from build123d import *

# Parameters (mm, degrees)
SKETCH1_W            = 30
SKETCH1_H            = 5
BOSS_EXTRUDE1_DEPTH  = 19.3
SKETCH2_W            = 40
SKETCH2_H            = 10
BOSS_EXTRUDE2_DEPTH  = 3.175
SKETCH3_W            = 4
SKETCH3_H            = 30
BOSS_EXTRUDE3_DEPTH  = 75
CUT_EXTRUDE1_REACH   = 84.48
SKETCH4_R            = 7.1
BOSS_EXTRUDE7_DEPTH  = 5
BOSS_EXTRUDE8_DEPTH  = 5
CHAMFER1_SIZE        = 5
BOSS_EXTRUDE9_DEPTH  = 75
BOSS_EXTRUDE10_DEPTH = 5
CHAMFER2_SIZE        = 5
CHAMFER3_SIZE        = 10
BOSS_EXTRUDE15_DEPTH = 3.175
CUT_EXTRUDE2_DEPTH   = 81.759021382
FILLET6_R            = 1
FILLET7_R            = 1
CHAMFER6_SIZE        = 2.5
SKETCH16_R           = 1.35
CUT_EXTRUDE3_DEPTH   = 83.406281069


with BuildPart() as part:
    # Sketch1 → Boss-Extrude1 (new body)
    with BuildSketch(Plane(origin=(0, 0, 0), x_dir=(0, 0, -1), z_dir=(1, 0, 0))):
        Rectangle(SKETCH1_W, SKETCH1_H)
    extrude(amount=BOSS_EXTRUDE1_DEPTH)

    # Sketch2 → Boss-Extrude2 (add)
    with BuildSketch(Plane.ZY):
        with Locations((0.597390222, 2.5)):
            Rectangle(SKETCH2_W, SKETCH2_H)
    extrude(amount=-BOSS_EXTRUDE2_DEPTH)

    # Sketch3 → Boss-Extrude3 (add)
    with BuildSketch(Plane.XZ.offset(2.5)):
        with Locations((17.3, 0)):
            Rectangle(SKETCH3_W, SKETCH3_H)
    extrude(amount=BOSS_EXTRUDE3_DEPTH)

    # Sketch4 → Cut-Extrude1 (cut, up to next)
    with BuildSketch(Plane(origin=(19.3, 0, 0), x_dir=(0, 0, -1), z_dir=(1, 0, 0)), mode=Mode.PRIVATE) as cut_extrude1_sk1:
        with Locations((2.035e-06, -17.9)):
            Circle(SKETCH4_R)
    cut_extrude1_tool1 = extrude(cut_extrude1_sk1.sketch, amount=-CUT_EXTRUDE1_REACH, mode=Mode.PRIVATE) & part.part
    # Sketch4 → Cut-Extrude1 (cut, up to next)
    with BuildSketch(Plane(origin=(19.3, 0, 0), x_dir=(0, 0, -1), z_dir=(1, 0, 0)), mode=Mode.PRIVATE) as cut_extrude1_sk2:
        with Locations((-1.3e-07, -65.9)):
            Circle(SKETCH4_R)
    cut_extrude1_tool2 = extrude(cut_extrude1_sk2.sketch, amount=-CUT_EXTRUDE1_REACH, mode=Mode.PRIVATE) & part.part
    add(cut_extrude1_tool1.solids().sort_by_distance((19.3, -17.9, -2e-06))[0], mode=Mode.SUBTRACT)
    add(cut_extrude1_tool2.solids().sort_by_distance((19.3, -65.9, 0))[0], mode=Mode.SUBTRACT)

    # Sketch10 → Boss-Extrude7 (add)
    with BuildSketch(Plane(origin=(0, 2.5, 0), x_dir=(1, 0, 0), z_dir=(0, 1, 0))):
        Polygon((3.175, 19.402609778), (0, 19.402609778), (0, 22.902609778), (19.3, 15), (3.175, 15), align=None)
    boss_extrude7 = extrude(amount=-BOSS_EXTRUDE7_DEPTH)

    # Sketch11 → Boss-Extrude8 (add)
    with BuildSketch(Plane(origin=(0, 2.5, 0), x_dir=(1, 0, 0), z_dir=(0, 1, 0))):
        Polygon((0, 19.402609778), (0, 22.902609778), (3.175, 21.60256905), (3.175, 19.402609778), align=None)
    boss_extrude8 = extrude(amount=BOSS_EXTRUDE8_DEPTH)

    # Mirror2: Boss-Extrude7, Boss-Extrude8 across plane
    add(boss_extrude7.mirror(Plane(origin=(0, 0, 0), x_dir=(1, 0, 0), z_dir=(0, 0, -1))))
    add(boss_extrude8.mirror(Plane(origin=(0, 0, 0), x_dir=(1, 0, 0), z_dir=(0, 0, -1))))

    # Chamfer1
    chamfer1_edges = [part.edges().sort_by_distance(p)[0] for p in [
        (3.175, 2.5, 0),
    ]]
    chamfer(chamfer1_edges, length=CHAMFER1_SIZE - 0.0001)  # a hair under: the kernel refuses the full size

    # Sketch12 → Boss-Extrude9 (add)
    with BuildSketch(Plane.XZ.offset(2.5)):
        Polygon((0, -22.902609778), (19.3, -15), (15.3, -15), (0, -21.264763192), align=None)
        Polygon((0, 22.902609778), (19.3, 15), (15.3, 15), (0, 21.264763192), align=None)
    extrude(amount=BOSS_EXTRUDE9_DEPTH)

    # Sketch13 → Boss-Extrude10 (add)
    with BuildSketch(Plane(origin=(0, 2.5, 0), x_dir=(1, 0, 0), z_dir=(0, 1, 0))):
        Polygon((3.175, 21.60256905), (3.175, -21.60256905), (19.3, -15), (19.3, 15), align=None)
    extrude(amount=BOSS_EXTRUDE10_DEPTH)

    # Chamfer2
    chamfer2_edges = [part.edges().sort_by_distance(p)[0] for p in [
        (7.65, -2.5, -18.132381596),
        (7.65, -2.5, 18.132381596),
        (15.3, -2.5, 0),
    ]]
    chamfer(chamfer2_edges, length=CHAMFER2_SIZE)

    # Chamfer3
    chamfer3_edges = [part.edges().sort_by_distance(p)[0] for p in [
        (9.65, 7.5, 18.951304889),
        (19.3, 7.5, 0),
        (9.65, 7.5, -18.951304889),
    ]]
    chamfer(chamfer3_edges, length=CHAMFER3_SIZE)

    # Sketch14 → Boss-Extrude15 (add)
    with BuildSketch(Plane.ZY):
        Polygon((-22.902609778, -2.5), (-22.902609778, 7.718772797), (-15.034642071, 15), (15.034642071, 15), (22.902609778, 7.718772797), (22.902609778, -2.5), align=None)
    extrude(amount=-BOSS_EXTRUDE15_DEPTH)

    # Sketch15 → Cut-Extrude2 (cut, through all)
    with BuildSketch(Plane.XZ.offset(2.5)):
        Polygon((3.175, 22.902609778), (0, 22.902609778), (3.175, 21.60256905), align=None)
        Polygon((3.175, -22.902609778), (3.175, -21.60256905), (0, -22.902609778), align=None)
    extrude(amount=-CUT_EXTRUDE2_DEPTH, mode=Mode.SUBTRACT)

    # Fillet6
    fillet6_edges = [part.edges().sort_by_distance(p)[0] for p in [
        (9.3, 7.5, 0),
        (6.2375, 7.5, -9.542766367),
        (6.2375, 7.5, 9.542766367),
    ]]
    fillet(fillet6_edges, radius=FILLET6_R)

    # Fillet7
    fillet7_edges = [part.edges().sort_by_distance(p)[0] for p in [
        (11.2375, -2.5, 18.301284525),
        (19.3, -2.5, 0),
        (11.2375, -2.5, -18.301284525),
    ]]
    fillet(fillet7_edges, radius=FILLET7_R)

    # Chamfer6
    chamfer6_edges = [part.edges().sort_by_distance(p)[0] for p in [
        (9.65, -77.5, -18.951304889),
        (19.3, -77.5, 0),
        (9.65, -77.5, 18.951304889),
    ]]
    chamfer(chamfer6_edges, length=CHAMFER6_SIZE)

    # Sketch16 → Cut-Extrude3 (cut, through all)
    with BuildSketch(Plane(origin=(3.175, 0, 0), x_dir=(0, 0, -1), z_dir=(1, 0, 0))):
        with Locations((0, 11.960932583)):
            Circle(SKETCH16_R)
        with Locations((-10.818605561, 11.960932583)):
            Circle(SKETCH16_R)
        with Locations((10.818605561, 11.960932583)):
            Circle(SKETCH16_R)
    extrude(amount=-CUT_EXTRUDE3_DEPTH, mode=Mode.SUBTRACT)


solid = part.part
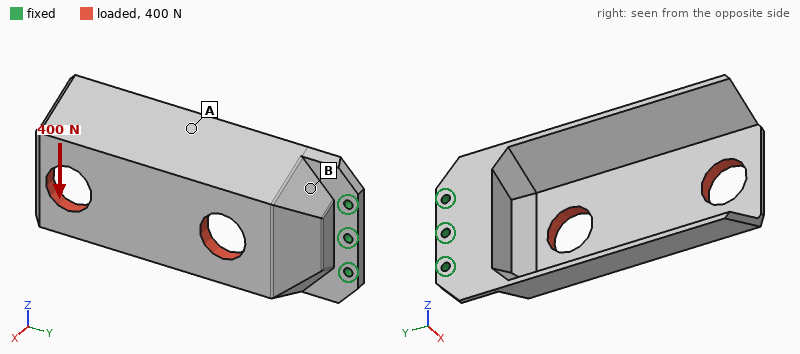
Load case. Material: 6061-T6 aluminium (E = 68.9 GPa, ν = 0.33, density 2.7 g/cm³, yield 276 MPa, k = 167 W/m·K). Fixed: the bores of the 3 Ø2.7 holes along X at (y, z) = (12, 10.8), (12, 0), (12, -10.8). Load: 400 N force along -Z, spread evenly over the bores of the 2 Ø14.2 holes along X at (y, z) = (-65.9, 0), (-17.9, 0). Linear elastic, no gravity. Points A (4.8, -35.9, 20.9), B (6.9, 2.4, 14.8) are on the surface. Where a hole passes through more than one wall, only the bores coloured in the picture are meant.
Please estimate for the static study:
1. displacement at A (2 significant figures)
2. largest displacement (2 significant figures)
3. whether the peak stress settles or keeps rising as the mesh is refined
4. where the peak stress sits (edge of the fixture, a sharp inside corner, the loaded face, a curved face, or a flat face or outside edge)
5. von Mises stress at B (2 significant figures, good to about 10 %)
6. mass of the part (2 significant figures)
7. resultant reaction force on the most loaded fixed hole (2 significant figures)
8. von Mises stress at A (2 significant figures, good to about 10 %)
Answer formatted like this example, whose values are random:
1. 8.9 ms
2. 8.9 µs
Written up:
1. 0.11 mm
2. 0.23 mm
3. keeps rising
4. edge of the fixture
5. 18 MPa
6. 49 g
7. 960 N
8. 6.5 MPa
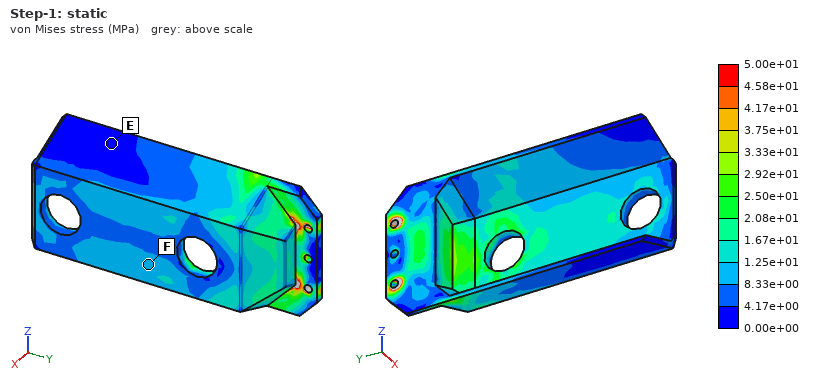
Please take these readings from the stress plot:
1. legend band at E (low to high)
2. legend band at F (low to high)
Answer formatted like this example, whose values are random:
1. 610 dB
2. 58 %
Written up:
1. 0.00e+00 to 4.17e+00 MPa
2. 8.33e+00 to 1.25e+01 MPa
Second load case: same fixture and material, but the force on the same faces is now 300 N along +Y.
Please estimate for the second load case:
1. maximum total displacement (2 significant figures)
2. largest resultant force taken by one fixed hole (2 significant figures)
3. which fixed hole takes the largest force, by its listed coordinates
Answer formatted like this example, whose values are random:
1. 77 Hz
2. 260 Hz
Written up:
1. 0.40 mm
2. 150 N
3. (12, 0)
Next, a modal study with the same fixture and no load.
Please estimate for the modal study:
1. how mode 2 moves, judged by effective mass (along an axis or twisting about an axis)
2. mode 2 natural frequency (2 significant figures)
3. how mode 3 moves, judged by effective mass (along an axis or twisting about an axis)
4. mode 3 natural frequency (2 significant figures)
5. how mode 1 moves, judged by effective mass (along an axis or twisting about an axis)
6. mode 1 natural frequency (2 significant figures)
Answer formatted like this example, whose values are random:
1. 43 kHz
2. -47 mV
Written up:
1. along Z
2. 1300 Hz
3. along Z
4. 3000 Hz
5. along X
6. 510 Hz
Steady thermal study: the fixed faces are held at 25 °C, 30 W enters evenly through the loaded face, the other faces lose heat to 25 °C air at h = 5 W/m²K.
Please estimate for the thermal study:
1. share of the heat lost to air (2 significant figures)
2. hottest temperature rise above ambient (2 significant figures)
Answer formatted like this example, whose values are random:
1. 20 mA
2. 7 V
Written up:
1. 7.4 %
2. 65 K
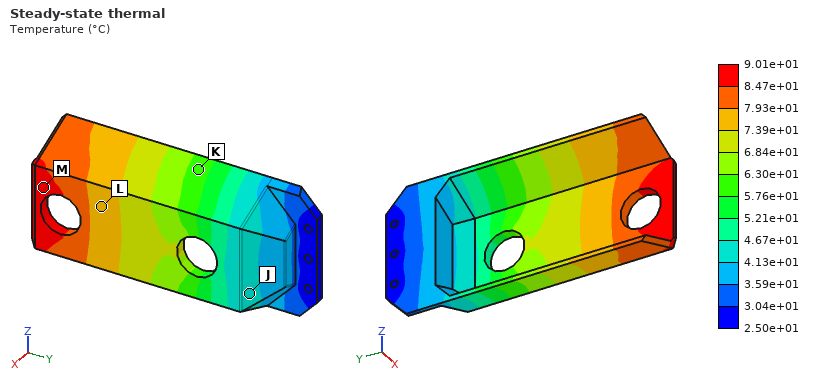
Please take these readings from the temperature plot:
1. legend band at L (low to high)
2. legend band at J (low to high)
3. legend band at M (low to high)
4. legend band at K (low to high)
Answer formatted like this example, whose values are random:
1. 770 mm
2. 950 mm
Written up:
1. 7.39e+01 to 7.93e+01 °C
2. 4.13e+01 to 4.67e+01 °C
3. 8.47e+01 to 9.01e+01 °C
4. 5.76e+01 to 6.30e+01 °C
